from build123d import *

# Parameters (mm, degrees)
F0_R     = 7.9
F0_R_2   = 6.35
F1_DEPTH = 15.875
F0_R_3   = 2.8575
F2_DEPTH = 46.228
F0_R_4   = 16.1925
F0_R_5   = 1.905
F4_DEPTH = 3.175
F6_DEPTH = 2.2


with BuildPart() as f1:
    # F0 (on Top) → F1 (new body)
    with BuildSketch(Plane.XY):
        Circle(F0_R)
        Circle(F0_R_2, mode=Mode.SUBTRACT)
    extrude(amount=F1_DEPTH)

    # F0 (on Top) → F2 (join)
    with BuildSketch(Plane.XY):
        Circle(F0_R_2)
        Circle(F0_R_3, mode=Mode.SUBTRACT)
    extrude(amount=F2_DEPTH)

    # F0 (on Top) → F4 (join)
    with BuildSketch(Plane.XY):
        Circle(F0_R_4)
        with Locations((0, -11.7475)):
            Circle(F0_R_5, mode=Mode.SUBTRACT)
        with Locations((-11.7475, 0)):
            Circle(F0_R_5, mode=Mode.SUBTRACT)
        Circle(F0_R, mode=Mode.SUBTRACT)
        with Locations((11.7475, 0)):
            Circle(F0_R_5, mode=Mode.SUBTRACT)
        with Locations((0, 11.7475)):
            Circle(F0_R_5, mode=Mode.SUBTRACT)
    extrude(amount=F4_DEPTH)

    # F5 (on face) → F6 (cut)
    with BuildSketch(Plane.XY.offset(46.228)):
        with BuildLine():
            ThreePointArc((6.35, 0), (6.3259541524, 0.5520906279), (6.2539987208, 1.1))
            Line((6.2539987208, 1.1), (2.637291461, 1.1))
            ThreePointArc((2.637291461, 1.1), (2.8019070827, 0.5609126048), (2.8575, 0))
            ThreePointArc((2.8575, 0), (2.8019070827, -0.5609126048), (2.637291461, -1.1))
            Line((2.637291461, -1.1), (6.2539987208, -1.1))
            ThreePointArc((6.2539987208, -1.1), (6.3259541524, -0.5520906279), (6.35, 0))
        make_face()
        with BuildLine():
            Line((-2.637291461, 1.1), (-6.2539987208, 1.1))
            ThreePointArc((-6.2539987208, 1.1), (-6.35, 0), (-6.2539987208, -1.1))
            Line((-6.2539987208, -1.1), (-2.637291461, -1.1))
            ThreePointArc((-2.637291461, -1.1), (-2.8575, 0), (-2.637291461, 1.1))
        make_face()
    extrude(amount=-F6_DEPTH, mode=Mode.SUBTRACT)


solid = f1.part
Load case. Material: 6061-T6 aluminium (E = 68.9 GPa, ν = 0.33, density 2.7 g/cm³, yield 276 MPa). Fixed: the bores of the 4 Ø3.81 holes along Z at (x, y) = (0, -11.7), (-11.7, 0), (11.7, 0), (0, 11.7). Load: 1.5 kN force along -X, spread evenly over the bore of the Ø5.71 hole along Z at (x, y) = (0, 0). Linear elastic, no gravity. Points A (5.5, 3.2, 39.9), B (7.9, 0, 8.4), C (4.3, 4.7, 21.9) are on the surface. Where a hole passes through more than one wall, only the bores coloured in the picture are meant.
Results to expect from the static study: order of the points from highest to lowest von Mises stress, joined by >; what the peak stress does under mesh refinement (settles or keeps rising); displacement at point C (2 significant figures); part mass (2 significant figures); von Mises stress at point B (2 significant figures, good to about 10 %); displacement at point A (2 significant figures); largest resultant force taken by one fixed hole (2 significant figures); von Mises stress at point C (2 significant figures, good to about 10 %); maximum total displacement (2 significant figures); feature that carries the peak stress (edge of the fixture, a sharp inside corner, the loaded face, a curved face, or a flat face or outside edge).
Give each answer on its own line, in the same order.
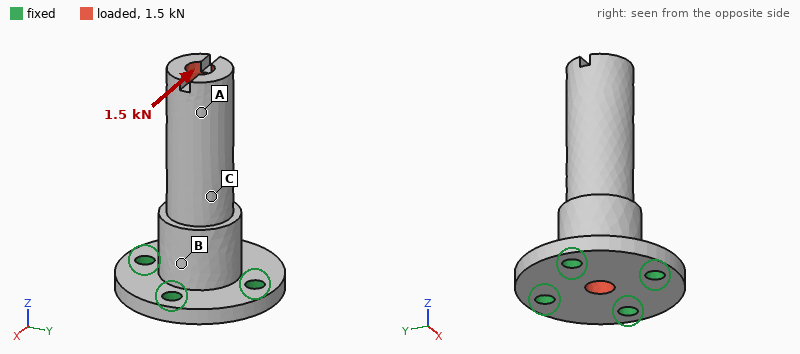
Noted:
B > C > A
keeps rising
0.063 mm
20 g
63 MPa
0.15 mm
1.7 kN
35 MPa
0.18 mm
edge of the fixture
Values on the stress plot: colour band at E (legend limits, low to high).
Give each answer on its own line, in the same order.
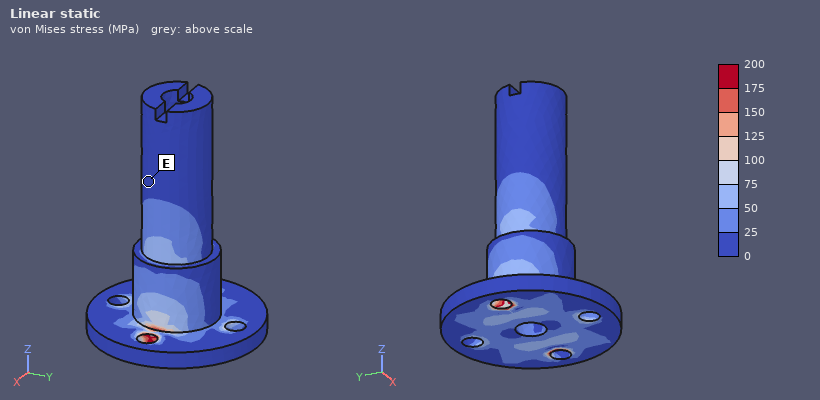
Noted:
0 to 25 MPa
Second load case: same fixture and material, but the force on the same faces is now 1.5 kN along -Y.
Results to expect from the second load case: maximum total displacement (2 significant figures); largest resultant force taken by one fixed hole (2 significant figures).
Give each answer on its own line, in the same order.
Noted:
0.18 mm
1.7 kN
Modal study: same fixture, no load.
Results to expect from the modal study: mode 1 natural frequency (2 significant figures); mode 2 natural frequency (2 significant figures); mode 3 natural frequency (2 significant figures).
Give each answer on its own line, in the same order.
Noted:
5000 Hz
5000 Hz
21 kHz
